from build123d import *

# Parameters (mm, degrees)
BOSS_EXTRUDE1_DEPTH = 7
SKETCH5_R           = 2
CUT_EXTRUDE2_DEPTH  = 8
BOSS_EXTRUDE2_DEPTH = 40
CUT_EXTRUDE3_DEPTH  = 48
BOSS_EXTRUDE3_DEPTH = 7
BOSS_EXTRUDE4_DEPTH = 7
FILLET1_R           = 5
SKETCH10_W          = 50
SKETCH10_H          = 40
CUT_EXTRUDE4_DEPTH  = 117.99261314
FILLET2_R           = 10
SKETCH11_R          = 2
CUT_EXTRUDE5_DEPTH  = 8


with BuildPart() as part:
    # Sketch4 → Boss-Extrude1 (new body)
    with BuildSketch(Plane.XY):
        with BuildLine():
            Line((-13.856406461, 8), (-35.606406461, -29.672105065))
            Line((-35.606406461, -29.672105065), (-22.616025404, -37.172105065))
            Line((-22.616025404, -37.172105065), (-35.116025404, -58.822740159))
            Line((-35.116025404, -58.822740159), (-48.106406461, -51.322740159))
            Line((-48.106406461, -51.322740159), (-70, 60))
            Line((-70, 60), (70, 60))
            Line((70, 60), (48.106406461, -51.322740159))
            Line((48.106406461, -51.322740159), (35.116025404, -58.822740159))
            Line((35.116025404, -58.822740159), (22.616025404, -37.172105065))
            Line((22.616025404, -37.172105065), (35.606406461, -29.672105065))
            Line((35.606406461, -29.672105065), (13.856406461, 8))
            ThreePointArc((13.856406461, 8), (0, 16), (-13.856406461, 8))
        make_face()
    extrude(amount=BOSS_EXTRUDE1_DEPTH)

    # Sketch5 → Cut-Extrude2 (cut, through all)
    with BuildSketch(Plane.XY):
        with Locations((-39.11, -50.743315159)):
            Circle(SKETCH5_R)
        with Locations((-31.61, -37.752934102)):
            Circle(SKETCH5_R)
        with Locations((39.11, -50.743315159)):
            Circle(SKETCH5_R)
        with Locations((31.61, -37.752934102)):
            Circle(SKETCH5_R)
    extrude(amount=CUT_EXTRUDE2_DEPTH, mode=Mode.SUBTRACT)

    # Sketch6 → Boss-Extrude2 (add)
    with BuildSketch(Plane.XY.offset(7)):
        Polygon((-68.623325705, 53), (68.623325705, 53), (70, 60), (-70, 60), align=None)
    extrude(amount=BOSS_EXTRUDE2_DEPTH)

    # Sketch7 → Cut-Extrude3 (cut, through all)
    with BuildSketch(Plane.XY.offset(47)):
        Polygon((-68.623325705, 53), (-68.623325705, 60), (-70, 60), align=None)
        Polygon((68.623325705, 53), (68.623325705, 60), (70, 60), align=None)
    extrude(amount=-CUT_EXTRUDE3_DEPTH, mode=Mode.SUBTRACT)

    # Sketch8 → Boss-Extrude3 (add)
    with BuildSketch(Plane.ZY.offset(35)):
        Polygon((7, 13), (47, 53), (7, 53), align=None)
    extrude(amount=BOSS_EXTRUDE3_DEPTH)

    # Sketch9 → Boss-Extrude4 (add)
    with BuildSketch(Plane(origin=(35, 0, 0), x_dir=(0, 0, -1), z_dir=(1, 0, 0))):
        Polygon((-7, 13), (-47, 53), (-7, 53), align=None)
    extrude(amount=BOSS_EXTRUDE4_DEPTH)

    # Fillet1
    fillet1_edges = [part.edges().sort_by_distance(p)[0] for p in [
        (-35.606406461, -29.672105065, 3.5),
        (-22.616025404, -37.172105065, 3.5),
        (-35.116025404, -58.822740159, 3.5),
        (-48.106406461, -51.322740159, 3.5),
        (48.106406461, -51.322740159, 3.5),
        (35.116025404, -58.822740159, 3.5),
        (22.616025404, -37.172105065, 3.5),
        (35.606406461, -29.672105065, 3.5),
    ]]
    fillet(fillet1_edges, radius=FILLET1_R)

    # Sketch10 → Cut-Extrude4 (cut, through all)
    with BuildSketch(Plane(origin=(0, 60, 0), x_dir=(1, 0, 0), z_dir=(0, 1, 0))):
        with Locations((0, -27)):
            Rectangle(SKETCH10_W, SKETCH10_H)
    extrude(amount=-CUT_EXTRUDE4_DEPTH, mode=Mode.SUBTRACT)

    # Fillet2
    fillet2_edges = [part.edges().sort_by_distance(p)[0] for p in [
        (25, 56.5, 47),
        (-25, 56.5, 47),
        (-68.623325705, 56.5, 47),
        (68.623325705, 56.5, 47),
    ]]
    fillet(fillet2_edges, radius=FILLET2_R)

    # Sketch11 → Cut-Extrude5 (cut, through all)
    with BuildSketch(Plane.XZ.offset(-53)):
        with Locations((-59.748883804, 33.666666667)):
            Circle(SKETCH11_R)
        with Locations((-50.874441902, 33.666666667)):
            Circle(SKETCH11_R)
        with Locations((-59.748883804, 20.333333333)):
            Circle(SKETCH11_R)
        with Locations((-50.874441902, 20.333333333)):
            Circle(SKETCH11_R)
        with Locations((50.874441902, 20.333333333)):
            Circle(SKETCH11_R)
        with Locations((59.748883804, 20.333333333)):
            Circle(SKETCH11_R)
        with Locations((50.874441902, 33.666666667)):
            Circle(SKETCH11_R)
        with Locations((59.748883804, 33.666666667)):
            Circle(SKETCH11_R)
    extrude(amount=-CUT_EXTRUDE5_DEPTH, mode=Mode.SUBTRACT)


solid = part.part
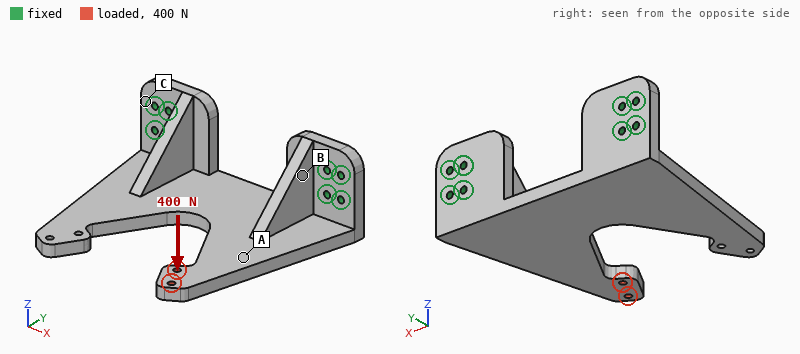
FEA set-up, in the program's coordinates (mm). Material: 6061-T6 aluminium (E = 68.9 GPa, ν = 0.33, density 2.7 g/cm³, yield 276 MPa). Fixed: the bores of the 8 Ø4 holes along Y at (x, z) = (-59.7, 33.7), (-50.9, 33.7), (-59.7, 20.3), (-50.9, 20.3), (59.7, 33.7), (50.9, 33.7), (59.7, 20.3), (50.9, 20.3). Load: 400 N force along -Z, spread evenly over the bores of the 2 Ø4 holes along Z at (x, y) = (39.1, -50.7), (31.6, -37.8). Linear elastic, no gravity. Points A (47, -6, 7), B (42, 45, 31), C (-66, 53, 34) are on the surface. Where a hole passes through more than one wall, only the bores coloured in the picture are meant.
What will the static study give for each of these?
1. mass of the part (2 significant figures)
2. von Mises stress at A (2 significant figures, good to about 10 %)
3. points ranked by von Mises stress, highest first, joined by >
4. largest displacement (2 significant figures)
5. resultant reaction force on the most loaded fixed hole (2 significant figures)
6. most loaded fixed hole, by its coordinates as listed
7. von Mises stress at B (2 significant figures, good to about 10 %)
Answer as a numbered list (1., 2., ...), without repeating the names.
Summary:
1. 280 g
2. 54 MPa
3. A > B > C
4. 0.87 mm
5. 1.5 kN
6. (50.9, 33.7)
7. 25 MPa
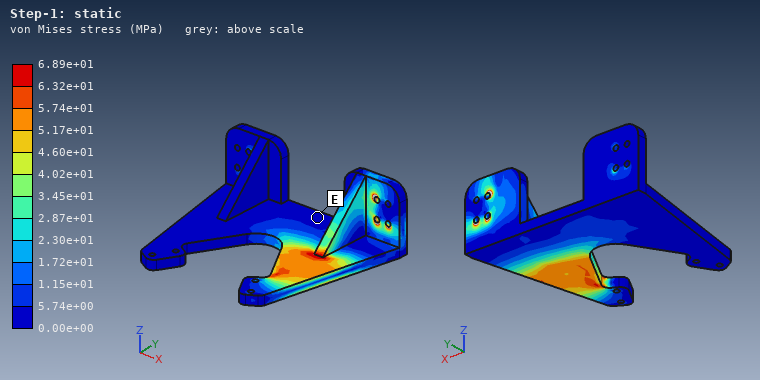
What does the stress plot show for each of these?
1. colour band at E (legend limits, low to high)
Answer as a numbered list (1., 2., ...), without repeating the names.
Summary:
1. 0.00e+00 to 5.74e+00 MPa
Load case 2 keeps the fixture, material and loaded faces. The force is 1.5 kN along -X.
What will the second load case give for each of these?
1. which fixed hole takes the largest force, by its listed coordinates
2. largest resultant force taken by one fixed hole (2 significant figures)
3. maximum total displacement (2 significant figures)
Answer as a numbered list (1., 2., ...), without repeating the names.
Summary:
1. (-50.9, 20.3)
2. 1.8 kN
3. 0.24 mm
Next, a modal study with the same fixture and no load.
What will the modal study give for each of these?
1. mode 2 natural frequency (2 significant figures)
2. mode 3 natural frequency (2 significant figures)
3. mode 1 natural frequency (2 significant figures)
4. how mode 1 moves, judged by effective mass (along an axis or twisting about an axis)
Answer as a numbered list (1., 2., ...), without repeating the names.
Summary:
1. 1100 Hz
2. 2700 Hz
3. 1000 Hz
4. along Z
